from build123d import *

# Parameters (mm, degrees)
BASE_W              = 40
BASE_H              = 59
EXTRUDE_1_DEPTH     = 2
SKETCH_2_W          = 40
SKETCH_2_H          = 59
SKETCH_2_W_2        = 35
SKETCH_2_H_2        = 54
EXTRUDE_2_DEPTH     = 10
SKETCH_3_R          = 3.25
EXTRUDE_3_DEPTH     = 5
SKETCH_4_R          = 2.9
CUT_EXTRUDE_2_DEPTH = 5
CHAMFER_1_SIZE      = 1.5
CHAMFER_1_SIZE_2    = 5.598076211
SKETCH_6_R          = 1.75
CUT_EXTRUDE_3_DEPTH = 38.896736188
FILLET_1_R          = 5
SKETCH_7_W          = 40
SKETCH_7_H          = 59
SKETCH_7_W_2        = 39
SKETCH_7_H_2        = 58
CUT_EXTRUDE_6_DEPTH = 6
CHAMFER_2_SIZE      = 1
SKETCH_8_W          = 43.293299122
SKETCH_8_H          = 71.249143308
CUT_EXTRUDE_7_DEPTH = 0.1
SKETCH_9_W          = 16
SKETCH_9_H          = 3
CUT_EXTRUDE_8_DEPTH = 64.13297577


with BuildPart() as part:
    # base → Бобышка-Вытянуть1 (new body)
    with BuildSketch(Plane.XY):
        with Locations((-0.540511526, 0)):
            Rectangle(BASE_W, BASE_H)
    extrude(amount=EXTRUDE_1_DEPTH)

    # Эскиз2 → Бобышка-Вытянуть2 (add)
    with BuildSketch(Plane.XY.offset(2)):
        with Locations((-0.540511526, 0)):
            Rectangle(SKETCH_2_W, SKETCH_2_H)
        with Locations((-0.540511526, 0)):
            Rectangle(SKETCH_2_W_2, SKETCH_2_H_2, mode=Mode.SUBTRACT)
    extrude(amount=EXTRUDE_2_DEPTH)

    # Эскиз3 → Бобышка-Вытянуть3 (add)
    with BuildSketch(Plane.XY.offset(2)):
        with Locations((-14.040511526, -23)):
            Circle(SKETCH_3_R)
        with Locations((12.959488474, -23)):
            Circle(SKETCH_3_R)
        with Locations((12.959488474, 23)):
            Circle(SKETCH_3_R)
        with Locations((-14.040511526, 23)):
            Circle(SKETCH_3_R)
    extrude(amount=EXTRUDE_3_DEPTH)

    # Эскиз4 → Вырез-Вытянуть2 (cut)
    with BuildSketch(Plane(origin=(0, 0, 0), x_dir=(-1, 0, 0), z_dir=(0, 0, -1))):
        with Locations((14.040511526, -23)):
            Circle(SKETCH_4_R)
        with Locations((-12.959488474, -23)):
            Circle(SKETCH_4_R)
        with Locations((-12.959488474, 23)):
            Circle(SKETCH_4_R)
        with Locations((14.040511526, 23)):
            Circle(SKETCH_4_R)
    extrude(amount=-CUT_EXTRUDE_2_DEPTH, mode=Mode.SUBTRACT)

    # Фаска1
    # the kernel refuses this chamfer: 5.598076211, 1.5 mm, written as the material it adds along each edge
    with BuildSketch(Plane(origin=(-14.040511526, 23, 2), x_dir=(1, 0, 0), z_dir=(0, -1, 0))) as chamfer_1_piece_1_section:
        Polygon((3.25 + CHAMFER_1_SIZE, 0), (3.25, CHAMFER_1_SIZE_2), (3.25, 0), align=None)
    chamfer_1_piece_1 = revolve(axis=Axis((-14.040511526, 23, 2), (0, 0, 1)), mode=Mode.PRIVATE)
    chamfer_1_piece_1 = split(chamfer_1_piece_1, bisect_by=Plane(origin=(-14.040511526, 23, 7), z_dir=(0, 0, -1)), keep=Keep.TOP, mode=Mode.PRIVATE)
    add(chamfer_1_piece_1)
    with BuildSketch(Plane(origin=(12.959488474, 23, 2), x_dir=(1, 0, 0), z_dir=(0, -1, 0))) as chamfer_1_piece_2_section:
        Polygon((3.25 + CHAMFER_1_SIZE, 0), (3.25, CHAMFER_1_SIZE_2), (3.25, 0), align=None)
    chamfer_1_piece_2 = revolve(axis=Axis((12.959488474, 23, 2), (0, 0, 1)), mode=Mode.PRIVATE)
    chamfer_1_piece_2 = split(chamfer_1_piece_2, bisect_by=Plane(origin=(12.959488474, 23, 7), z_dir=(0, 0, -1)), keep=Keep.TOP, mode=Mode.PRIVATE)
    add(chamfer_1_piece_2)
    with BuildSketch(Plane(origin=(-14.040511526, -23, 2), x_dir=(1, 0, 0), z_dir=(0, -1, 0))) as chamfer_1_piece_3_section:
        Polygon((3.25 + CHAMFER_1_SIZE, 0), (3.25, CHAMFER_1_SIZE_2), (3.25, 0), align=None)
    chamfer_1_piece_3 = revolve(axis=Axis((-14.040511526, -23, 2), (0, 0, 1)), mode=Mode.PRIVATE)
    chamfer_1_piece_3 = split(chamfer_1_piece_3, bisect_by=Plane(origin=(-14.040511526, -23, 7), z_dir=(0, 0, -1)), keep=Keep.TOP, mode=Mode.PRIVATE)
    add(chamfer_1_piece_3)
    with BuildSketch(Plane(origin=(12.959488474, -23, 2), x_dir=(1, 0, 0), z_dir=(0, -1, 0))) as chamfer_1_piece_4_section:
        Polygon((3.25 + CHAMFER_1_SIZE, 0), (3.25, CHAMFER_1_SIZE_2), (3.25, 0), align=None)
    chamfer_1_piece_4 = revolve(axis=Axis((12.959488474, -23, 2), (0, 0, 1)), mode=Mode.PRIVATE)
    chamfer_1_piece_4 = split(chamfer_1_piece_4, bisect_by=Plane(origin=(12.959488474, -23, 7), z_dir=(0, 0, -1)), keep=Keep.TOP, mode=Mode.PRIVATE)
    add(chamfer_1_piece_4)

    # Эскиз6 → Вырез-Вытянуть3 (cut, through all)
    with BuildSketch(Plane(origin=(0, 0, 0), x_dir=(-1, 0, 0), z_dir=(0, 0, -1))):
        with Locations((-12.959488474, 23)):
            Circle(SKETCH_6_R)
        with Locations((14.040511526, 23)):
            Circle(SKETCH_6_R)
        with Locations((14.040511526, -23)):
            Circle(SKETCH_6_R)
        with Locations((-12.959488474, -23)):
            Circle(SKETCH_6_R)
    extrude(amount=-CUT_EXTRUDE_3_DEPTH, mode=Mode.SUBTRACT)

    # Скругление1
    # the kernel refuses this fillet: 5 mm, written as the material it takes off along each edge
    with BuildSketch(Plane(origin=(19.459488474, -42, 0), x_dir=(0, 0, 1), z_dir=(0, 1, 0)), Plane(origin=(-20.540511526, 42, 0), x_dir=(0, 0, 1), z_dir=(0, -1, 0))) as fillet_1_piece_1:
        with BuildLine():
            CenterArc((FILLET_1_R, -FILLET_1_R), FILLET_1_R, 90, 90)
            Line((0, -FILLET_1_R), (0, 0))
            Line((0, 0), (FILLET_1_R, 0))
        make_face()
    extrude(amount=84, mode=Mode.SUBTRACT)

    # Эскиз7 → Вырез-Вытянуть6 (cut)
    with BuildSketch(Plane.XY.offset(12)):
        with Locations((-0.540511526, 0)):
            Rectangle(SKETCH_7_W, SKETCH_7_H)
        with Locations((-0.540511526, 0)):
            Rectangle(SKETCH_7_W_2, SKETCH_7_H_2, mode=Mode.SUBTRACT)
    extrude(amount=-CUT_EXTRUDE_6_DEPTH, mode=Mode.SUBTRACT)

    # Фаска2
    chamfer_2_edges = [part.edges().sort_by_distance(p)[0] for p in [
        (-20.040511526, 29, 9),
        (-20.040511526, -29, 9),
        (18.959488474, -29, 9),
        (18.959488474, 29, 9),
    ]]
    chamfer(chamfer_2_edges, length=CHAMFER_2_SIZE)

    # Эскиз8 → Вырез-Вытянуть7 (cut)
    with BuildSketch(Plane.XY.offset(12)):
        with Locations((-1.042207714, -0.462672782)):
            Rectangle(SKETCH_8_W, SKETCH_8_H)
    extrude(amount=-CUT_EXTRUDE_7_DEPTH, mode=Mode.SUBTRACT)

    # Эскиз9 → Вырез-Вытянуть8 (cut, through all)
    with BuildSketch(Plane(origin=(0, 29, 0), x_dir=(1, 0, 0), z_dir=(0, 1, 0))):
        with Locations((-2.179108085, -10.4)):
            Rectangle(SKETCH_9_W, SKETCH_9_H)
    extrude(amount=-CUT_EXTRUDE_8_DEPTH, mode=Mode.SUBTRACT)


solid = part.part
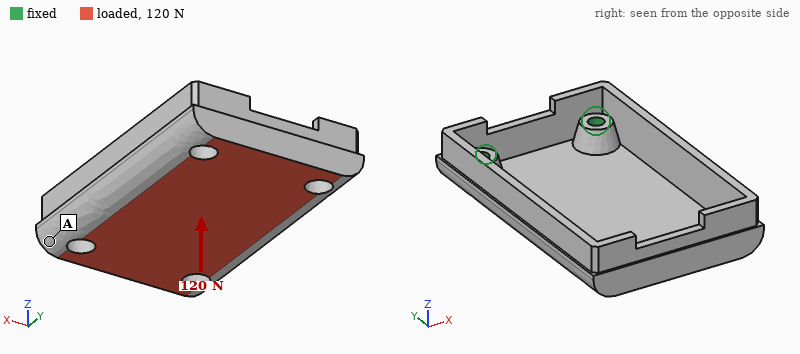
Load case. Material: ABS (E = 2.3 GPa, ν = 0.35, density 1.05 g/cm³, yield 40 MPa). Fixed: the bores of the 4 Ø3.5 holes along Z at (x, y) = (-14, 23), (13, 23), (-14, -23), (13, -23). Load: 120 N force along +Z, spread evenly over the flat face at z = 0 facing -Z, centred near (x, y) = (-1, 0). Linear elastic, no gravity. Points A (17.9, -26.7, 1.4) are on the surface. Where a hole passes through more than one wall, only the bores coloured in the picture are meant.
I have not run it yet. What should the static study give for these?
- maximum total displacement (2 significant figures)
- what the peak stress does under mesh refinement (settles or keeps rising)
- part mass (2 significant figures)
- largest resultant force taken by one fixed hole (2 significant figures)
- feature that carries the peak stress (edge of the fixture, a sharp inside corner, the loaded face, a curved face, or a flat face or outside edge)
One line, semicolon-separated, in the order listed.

0.26 mm; keeps rising; 8.8 g; 35 N; edge of the fixture
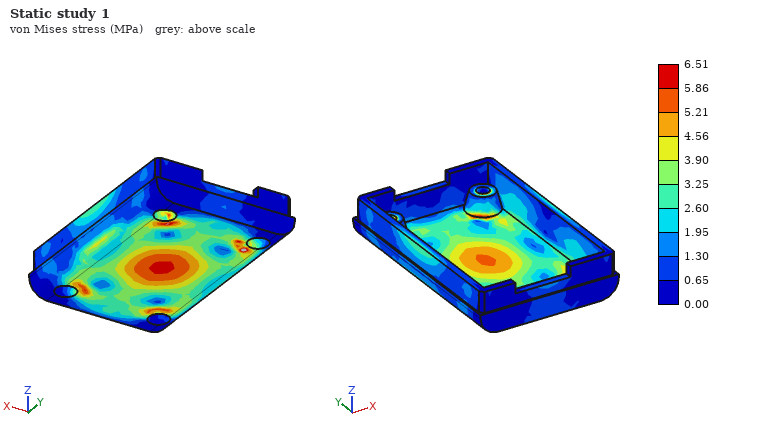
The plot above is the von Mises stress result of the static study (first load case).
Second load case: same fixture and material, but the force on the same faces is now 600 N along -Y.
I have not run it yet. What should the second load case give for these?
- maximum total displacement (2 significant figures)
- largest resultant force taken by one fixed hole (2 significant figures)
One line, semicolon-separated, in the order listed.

0.12 mm; 150 N
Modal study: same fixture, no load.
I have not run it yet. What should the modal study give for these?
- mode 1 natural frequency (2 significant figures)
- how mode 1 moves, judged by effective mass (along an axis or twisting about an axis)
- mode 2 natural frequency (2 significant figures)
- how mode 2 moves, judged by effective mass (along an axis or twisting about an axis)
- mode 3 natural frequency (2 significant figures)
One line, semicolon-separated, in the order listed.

2100 Hz; along Z; 2700 Hz; along X; 2900 Hz
